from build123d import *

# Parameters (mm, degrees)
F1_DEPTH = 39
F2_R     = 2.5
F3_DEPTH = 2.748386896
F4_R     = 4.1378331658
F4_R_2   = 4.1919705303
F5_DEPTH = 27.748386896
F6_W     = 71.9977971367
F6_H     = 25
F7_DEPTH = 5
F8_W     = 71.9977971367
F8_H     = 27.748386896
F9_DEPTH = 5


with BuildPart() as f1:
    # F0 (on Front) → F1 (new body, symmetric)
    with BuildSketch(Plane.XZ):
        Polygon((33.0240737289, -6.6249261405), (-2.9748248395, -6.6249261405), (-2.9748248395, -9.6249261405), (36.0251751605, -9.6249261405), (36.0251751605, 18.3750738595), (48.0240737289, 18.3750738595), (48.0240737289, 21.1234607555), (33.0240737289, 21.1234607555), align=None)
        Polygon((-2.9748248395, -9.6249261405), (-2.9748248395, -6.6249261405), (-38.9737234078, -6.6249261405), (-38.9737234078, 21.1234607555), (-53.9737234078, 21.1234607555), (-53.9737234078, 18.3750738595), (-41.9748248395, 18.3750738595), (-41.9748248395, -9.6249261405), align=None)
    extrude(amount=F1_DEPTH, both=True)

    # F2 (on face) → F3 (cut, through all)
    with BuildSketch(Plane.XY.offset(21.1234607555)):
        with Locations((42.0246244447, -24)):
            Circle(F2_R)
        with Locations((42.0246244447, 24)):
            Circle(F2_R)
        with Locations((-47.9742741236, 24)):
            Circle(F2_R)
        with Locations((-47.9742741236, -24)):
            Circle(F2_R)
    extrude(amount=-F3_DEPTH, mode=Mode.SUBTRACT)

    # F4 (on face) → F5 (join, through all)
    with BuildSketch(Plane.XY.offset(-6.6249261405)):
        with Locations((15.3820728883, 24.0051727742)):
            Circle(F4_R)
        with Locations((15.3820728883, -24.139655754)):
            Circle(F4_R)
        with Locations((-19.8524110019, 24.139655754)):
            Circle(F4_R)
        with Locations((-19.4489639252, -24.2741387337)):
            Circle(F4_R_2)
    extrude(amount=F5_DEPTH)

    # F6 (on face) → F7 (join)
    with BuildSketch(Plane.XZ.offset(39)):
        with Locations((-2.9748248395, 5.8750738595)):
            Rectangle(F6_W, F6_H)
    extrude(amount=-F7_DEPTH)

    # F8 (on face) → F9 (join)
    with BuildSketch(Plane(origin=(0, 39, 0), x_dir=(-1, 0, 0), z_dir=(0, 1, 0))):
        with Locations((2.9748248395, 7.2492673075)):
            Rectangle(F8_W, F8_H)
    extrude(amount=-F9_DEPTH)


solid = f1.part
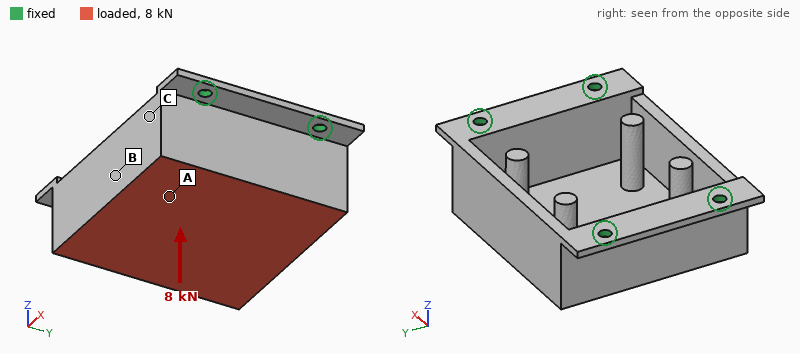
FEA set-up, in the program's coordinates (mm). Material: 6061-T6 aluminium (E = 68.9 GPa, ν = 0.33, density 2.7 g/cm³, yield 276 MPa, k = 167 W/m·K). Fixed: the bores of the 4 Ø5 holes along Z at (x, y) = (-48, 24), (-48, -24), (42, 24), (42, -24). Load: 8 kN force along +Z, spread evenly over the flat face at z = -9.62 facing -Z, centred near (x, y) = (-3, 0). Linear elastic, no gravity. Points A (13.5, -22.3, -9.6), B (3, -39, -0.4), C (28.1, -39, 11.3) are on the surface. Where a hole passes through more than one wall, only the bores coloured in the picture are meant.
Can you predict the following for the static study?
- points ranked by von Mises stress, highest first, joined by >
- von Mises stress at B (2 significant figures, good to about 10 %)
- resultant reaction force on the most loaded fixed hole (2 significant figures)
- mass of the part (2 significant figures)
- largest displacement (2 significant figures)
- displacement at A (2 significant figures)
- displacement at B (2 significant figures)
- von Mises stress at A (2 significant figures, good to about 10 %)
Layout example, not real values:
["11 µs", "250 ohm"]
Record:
["A > B > C", "31 MPa", "2.1 kN", "170 g", "0.41 mm", "0.18 mm", "0.070 mm", "55 MPa"]
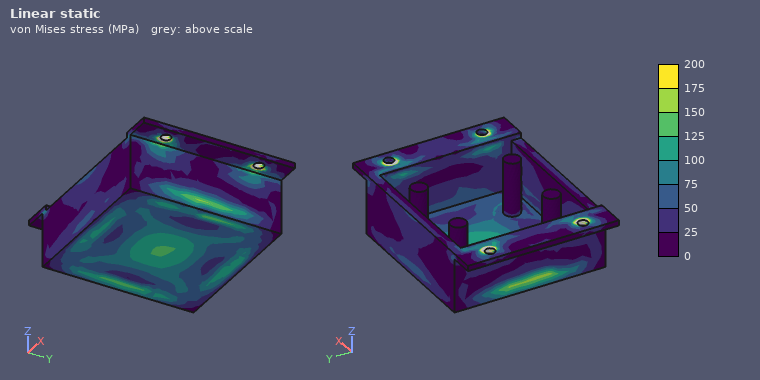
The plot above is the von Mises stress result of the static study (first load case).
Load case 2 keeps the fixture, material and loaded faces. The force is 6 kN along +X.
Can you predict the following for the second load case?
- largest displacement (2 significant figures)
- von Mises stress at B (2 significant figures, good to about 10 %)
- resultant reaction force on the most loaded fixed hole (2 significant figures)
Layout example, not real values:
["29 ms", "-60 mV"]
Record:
["74 µm", "24 MPa", "2.1 kN"]
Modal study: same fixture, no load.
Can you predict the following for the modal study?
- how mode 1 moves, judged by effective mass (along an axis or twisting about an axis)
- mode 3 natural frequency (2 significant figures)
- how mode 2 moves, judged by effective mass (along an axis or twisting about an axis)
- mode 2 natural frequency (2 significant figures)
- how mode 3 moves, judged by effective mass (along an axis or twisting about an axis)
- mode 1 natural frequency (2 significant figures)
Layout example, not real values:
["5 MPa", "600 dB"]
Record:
["along Z", "4100 Hz", "along Y", "3200 Hz", "along X", "3000 Hz"]
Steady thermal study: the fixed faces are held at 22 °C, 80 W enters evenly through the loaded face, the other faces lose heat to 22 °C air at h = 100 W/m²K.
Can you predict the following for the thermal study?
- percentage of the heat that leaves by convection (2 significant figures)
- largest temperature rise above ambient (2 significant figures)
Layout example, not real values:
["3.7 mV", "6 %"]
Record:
["53 %", "26 K"]
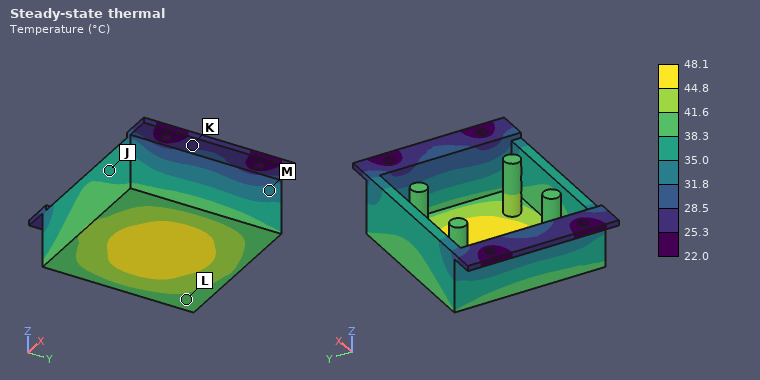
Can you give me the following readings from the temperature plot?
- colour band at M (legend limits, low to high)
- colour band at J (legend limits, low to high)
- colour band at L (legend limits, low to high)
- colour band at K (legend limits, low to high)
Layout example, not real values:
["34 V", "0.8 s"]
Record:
["31.8 to 35.0 °C", "35.0 to 38.3 °C", "38.3 to 41.6 °C", "25.3 to 28.5 °C"]
